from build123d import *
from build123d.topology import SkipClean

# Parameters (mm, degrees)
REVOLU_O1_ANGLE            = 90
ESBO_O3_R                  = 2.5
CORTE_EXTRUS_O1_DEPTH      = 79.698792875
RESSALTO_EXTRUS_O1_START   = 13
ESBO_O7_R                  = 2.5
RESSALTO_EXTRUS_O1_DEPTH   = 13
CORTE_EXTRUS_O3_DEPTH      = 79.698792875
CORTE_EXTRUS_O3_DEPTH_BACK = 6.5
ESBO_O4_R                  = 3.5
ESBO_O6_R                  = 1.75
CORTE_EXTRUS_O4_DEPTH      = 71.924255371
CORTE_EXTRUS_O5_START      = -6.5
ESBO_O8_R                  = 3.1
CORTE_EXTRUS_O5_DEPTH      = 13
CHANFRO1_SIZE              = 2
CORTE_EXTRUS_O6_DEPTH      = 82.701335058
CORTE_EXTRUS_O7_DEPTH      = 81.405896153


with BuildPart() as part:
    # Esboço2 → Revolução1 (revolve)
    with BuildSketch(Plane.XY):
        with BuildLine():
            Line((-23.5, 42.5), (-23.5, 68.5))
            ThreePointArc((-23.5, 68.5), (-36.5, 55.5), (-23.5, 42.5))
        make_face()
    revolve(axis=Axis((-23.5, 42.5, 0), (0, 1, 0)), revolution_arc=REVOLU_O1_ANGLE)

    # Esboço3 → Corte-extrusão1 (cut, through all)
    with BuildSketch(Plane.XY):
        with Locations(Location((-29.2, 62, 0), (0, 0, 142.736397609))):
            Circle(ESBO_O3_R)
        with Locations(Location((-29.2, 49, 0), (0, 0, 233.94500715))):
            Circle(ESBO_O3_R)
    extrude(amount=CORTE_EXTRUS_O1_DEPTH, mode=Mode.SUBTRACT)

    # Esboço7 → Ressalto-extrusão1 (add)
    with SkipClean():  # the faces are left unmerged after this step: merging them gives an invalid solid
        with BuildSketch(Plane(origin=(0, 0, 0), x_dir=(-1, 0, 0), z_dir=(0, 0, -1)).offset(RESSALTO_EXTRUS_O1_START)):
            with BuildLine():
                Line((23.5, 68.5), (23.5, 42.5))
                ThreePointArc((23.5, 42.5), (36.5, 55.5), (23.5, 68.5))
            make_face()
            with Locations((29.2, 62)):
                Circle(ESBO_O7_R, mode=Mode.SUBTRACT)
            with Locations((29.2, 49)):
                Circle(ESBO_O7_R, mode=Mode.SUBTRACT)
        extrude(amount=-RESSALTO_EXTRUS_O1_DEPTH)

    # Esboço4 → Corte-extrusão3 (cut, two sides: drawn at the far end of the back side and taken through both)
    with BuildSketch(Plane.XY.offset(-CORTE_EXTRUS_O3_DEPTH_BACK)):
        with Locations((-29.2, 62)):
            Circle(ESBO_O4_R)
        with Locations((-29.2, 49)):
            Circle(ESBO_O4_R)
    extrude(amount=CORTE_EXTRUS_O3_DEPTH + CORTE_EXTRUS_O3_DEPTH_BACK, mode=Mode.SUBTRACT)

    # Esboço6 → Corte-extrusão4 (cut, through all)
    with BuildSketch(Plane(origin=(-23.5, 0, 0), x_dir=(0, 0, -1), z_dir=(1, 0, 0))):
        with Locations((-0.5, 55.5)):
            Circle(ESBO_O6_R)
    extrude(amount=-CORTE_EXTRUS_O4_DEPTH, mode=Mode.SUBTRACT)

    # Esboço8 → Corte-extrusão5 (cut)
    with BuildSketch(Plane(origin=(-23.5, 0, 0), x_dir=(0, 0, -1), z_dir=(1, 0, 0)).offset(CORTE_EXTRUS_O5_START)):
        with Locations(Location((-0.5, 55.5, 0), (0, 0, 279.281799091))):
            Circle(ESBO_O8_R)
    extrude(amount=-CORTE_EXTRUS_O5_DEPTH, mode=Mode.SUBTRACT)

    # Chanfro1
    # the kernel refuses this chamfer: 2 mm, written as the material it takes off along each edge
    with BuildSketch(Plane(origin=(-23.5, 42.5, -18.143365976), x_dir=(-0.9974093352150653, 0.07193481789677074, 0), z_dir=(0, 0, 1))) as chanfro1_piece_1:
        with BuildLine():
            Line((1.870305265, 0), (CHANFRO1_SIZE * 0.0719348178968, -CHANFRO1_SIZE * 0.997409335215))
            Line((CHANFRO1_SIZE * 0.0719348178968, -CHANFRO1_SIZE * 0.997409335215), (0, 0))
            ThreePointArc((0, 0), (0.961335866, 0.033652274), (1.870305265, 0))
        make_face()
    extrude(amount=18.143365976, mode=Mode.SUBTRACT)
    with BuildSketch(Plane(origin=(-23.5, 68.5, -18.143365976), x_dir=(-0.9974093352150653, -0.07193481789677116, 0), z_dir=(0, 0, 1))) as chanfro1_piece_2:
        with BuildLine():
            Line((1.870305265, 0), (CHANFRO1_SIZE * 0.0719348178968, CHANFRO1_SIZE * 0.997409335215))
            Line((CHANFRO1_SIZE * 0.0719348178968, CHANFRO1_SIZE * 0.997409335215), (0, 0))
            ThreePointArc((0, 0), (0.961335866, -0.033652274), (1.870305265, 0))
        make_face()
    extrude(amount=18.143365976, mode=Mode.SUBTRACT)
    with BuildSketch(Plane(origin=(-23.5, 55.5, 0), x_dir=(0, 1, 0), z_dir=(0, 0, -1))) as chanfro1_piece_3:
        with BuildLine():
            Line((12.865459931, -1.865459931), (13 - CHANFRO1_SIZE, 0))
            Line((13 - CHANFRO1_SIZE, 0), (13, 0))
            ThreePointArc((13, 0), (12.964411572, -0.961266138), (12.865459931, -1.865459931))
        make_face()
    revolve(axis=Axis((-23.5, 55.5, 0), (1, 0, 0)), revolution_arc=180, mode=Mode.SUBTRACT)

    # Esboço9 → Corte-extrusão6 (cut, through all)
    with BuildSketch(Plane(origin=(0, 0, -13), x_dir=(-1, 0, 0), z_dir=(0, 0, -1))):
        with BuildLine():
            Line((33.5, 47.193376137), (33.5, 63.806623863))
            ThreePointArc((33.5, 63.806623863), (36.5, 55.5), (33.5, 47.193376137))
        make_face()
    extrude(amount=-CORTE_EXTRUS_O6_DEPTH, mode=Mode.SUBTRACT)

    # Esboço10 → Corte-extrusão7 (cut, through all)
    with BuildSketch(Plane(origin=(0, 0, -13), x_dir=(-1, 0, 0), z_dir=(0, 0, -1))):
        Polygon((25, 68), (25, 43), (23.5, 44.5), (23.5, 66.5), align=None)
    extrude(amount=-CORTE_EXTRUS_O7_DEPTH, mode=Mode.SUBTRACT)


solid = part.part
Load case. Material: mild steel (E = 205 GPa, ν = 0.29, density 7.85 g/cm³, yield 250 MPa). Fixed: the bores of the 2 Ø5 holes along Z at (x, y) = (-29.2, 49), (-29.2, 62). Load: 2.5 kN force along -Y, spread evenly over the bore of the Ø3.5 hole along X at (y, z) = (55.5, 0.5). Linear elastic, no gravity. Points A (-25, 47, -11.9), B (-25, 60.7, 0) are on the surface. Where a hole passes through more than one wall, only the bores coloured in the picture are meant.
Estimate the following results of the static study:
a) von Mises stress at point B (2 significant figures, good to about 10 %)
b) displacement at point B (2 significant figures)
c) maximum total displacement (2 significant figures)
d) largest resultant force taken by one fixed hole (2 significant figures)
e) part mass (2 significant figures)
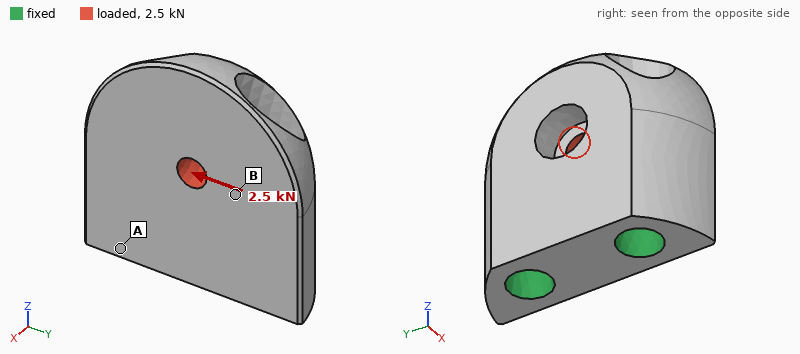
95 MPa
4.9 µm
7.7 µm
1.9 kN
21 g
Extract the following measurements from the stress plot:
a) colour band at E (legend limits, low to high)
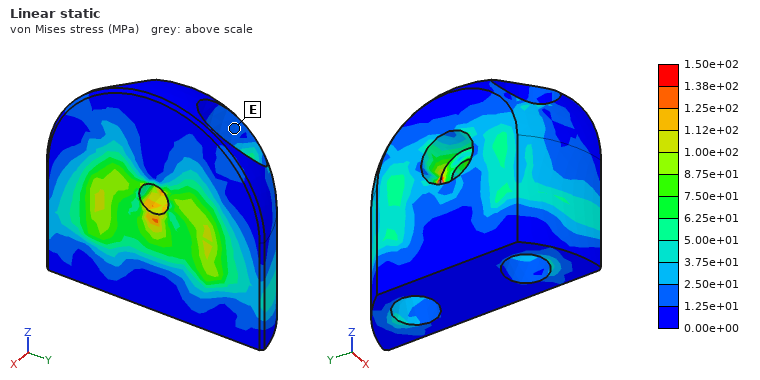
1.25e+01 to 2.50e+01 MPa
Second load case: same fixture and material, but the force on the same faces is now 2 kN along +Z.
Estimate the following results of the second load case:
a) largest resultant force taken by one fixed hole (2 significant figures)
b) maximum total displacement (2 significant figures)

1.0 kN
4.5 µm
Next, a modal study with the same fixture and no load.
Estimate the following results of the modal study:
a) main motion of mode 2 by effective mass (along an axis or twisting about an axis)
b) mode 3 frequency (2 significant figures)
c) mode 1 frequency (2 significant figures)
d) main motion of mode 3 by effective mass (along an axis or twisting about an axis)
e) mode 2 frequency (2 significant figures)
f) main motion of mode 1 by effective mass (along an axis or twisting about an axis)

along Y
34 kHz
15 kHz
twisting about Z
27 kHz
along X
